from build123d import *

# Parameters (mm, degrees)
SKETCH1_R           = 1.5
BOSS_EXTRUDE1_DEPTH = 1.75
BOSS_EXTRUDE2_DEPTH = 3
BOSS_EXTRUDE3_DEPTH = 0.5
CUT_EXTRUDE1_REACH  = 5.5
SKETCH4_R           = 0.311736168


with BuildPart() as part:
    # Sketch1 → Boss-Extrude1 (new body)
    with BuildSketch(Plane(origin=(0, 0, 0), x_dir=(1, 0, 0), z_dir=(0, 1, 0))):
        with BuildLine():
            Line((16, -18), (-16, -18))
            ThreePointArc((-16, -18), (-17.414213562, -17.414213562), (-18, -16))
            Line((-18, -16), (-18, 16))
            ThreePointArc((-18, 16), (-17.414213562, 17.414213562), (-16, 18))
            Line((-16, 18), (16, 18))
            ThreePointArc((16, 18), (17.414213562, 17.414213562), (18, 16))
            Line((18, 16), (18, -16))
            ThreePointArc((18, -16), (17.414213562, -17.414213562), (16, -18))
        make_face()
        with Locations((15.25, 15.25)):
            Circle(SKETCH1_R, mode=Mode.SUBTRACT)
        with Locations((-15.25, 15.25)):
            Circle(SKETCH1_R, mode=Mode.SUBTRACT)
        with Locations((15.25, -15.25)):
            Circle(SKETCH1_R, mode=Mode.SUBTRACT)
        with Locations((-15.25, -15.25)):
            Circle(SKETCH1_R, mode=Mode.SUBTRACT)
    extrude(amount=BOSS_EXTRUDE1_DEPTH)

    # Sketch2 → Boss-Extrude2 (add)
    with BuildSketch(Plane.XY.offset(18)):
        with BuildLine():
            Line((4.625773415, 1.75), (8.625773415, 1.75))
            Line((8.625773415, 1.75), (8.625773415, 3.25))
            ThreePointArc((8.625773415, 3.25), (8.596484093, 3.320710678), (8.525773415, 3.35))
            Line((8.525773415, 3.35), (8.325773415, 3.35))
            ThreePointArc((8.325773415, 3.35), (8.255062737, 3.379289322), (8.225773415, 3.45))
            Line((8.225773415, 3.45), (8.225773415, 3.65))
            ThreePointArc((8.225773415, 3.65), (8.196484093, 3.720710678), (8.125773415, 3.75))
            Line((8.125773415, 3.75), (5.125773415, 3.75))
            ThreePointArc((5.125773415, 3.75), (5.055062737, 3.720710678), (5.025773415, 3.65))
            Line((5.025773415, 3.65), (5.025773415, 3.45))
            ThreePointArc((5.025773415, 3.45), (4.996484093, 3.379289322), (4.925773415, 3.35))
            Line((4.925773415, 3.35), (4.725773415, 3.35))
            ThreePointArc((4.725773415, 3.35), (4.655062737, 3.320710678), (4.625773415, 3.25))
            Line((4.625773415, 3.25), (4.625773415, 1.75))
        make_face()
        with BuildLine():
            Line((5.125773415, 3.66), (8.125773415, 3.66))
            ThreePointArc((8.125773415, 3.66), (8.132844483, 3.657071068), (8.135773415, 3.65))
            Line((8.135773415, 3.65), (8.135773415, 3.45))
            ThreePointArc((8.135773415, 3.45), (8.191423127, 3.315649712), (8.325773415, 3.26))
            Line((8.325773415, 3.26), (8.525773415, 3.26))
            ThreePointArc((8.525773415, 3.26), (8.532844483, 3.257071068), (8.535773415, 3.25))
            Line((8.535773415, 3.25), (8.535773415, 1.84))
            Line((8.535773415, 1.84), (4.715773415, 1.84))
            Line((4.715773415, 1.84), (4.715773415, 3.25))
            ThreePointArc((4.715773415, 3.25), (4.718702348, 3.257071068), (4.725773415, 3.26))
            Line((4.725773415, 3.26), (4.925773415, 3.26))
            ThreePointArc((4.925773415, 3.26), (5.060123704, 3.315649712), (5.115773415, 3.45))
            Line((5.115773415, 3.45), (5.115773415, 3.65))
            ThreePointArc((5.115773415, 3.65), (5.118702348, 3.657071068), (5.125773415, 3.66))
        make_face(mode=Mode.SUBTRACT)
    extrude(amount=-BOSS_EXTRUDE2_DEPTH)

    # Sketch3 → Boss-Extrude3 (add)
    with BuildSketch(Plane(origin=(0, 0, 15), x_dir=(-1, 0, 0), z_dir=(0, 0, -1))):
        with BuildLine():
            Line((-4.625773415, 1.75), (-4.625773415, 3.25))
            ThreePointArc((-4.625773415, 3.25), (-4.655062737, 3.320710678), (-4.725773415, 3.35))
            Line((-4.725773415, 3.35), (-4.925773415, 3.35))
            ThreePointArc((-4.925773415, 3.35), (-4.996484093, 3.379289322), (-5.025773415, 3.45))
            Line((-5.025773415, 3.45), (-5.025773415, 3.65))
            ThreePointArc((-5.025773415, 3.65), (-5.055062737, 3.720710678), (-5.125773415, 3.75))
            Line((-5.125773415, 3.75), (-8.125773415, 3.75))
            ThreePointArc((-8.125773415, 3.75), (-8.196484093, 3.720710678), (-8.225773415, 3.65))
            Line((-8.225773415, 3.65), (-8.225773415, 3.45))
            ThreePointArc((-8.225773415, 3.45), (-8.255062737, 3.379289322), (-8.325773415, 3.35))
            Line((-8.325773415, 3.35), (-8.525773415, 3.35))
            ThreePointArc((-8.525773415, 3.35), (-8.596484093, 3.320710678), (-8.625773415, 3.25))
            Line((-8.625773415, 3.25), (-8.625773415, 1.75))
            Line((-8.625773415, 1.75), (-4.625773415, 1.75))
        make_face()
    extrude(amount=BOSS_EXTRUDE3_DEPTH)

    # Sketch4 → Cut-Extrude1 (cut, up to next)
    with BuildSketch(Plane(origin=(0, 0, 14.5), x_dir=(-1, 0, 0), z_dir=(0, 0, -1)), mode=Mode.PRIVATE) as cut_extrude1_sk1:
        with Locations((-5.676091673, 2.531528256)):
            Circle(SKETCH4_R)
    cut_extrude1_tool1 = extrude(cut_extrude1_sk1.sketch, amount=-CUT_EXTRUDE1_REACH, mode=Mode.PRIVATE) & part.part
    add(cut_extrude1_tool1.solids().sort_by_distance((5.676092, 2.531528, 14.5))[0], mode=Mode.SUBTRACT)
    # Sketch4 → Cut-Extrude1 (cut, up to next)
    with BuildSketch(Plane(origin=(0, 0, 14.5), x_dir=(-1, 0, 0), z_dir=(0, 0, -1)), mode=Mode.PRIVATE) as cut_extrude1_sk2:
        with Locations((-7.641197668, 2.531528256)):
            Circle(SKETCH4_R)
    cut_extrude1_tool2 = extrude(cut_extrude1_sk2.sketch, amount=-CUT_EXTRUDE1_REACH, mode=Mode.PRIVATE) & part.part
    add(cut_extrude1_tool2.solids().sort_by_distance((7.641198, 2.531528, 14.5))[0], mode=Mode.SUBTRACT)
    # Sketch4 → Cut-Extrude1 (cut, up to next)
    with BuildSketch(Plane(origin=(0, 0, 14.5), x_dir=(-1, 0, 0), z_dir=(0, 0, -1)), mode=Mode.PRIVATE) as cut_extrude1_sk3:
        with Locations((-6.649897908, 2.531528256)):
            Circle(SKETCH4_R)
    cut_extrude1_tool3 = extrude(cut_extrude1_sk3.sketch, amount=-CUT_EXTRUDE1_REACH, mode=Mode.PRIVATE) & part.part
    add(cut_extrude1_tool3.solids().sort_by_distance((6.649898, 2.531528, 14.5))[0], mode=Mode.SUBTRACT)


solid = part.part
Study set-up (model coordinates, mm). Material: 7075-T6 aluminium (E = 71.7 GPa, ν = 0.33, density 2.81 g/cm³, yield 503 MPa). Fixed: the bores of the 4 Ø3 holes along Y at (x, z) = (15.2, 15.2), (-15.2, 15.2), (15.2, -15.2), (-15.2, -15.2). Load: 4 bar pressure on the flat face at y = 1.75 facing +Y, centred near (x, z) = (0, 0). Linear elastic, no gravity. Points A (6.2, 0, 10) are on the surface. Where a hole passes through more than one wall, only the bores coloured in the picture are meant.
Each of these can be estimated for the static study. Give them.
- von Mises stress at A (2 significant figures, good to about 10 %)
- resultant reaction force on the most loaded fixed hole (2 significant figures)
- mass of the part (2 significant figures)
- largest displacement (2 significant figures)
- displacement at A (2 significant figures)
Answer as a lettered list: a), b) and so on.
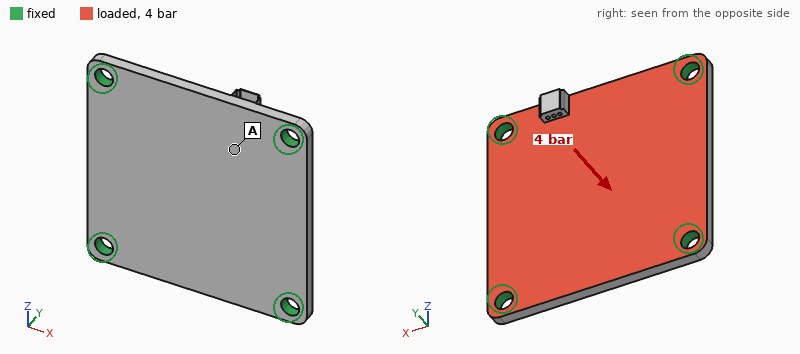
a) 19 MPa
b) 130 N
c) 6.2 g
d) 62 µm
e) 36 µm
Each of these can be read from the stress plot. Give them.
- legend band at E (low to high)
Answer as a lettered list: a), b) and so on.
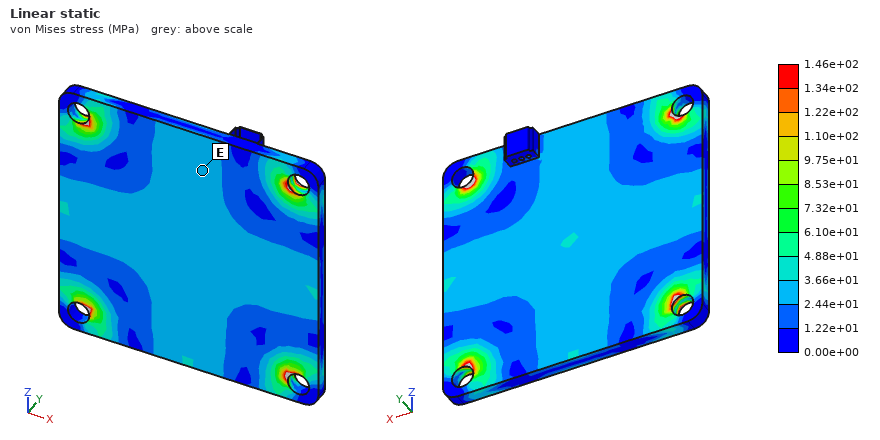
a) 2.44e+01 to 3.66e+01 MPa
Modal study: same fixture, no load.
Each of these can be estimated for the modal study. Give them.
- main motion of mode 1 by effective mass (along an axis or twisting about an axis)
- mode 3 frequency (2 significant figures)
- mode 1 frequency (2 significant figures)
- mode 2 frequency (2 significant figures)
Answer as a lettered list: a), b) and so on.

a) along Y
b) 12 kHz
c) 7000 Hz
d) 12 kHz
